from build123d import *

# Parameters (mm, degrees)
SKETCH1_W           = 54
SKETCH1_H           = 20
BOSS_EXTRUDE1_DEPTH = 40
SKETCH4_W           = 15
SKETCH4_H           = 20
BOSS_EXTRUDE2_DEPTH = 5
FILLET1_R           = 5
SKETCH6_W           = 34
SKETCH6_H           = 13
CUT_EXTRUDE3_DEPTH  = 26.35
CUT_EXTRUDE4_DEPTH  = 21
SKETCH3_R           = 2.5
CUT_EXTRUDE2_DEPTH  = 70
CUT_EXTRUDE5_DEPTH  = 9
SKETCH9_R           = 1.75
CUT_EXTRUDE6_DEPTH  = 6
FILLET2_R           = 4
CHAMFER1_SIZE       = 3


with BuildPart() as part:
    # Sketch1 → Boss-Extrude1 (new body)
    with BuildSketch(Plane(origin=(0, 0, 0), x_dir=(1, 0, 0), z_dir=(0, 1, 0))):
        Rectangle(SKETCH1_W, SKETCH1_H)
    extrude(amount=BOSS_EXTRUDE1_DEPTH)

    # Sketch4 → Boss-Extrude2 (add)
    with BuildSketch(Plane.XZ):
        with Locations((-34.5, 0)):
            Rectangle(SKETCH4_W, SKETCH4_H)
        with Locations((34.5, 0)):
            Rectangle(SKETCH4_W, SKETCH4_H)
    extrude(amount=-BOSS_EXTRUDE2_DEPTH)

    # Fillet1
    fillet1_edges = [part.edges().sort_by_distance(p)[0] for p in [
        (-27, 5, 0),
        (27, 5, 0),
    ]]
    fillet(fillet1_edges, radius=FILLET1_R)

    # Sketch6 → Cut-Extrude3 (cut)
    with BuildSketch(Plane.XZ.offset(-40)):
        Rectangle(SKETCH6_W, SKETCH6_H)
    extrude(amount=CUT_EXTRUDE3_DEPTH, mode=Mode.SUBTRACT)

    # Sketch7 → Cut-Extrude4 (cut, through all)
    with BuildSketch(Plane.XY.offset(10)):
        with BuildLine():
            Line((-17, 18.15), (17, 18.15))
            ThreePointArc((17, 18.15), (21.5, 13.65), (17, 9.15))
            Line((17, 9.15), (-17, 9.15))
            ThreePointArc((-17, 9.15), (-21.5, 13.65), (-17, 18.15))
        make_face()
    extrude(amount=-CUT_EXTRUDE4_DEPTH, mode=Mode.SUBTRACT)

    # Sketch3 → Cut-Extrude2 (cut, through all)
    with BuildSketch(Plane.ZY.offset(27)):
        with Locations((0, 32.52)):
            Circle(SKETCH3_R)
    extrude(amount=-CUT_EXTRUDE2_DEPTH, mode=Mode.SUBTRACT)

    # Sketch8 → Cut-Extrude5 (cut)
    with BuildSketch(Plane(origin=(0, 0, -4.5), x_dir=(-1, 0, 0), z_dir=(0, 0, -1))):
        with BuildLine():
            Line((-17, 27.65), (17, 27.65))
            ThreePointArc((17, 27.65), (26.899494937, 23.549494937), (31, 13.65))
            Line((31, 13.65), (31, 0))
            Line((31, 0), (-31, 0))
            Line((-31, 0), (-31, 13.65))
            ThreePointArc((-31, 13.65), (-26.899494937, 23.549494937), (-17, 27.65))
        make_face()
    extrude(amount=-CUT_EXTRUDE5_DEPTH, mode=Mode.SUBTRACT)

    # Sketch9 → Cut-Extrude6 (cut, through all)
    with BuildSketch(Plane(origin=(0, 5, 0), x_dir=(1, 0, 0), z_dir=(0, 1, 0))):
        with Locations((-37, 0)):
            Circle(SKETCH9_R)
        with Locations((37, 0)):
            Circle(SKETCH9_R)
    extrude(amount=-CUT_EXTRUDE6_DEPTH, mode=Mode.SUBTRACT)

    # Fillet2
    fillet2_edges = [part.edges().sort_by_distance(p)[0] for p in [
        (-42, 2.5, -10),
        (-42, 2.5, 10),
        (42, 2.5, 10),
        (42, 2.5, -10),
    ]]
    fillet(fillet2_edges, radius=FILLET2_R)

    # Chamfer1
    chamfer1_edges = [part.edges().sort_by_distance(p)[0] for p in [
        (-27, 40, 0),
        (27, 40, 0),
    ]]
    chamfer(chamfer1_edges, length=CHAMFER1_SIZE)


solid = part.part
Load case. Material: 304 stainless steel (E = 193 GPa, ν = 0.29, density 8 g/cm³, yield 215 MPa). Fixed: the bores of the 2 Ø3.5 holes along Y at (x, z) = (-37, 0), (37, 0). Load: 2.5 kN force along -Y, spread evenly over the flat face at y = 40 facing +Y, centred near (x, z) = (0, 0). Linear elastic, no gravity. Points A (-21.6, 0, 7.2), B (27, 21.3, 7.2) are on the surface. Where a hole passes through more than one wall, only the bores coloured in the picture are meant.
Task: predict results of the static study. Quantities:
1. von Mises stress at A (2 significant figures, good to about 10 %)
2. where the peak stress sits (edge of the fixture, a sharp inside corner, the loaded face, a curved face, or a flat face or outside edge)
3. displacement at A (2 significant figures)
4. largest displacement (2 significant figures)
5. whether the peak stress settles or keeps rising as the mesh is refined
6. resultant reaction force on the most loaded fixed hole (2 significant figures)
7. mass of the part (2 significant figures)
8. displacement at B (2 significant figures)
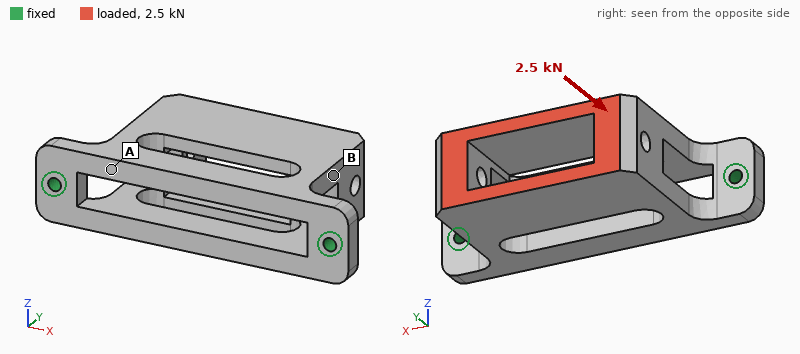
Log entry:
24 MPa
edge of the fixture
13 µm
17 µm
keeps rising
1.4 kN
170 g
14 µm
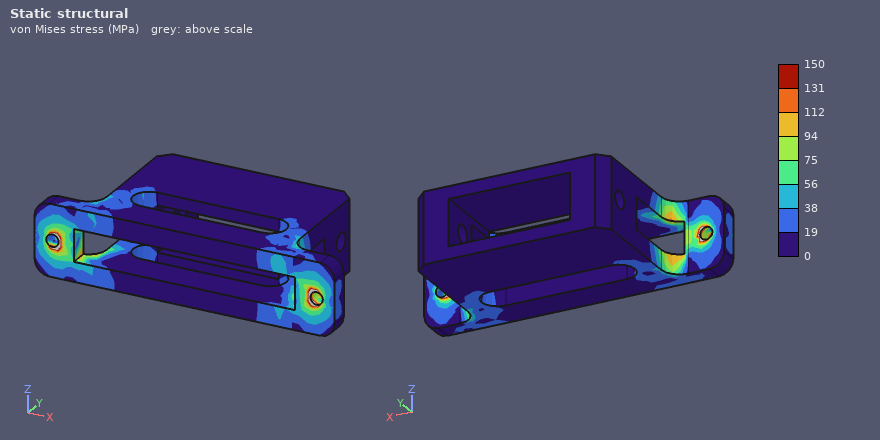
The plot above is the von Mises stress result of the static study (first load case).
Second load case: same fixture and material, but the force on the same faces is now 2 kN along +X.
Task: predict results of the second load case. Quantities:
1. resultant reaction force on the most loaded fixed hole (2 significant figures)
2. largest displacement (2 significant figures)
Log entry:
1.5 kN
23 µm
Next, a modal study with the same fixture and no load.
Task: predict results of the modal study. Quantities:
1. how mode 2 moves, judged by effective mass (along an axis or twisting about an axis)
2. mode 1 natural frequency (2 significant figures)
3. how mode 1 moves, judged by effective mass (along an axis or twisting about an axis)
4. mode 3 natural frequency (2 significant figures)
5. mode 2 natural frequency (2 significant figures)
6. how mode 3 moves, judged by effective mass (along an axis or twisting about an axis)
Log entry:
twisting about Y
1500 Hz
along Z
5100 Hz
4100 Hz
along Y
